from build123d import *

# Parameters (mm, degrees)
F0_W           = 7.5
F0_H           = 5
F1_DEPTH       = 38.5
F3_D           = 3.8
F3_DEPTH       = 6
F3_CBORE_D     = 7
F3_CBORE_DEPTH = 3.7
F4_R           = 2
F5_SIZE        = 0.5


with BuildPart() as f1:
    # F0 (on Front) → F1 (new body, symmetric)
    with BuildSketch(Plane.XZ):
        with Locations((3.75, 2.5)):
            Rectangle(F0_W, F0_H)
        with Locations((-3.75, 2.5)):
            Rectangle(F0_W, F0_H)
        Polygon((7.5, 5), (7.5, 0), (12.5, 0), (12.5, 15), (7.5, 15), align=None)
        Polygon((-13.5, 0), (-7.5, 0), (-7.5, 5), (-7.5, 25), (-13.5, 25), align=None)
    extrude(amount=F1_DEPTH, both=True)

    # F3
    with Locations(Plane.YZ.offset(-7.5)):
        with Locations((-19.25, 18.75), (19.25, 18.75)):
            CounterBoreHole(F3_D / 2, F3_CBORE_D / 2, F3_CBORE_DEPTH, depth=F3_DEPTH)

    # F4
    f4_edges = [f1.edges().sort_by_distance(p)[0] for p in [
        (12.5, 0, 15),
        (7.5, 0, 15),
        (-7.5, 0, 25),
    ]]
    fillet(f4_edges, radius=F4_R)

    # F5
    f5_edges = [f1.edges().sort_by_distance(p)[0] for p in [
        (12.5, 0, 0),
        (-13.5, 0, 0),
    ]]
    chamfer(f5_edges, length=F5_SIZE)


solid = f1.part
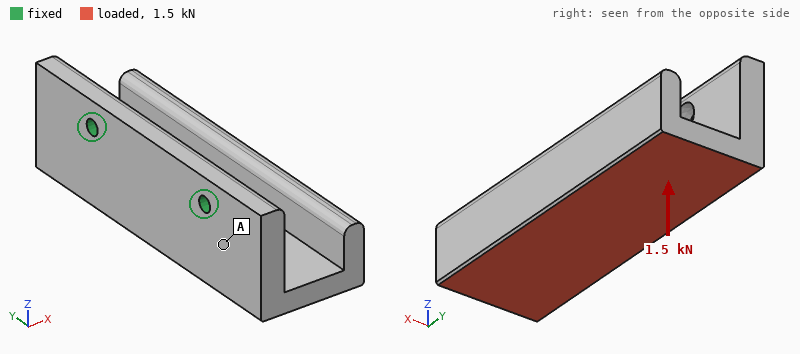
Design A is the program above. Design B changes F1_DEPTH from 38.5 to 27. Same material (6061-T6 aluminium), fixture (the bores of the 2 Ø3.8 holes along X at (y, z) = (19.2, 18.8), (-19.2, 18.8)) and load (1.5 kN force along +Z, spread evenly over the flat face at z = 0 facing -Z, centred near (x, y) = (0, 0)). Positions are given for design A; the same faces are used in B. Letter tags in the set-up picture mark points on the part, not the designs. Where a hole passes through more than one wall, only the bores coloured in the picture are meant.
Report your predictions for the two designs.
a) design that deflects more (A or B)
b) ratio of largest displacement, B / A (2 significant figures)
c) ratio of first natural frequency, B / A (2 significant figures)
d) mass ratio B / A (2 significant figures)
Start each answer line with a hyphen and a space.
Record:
- B
- 1.1
- 1.1
- 0.70
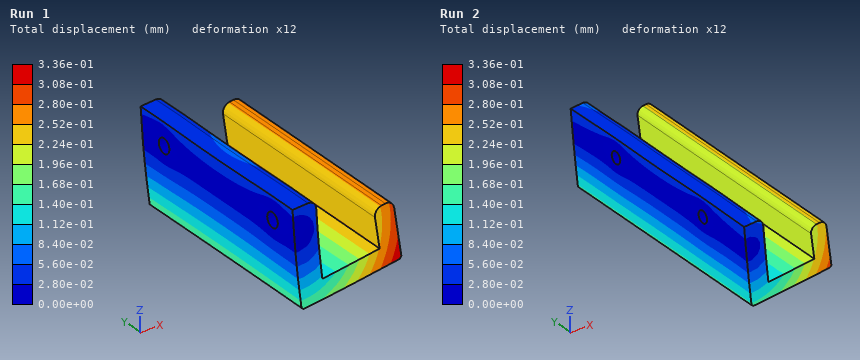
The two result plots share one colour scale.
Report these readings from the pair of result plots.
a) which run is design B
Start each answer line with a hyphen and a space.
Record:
- Run 1
